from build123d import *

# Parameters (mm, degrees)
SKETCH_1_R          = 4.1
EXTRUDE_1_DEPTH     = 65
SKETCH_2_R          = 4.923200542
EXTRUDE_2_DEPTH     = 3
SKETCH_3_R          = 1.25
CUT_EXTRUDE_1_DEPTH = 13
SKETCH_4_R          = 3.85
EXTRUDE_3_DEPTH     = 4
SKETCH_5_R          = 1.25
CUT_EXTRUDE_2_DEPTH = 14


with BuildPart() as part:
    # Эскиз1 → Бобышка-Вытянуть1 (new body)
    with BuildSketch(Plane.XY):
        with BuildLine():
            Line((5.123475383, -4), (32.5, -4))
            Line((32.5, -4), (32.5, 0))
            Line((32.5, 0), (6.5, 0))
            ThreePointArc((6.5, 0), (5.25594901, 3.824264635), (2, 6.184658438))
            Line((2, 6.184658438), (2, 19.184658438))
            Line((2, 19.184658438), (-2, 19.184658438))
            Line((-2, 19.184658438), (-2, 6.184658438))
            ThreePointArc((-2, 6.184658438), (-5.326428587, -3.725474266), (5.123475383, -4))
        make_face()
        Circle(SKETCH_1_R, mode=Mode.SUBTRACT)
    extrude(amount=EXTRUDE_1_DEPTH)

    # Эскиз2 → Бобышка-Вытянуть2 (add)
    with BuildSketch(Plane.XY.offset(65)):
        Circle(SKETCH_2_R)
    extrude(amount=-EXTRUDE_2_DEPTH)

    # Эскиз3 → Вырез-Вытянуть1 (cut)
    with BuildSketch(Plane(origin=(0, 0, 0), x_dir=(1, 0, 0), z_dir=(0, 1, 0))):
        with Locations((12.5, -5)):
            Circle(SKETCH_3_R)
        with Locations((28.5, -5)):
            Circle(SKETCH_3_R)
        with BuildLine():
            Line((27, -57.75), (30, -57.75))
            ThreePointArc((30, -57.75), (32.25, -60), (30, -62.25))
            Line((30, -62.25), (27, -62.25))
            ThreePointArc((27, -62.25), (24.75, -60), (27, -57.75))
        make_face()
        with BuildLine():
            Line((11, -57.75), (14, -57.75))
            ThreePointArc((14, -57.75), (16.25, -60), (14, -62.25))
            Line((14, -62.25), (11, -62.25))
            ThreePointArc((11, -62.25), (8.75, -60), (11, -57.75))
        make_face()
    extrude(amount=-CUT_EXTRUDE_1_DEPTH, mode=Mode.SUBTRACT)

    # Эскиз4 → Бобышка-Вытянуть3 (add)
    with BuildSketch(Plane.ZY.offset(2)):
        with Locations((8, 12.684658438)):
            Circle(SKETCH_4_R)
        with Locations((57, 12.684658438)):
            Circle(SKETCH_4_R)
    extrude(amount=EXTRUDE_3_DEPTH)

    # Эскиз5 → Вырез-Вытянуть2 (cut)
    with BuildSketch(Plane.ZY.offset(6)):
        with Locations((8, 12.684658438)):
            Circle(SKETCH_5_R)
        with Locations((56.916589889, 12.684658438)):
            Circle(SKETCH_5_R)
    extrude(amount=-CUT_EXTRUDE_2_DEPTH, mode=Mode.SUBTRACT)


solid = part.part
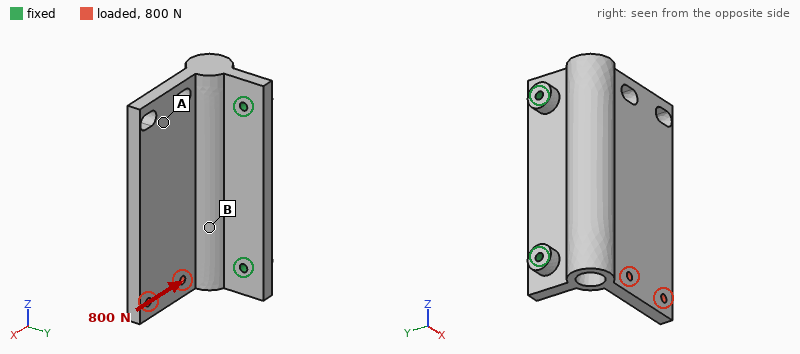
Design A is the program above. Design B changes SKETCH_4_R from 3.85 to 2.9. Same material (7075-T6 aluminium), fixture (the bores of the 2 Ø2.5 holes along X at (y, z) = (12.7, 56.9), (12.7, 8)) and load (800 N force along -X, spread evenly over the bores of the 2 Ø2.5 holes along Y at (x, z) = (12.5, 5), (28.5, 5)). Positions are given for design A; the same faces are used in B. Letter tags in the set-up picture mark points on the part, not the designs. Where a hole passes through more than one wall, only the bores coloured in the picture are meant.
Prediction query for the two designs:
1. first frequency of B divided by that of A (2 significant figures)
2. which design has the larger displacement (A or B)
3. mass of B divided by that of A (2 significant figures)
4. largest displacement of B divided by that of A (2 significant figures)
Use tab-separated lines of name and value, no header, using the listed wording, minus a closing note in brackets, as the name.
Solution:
first frequency of B divided by that of A	0.95
which design has the larger displacement	B
mass of B divided by that of A	0.99
largest displacement of B divided by that of A	1.1
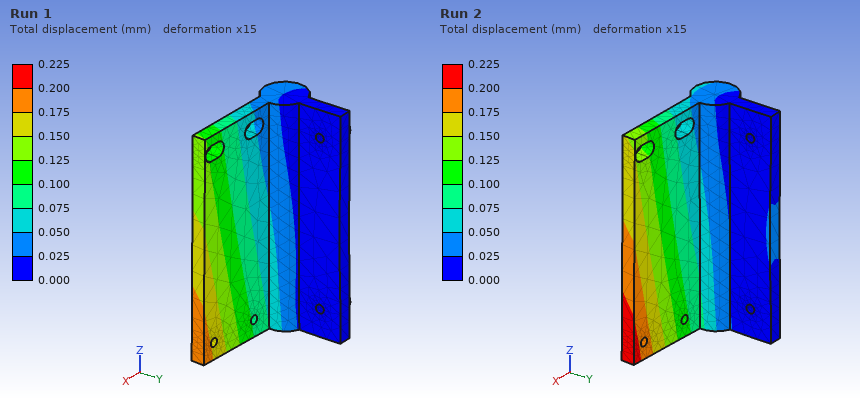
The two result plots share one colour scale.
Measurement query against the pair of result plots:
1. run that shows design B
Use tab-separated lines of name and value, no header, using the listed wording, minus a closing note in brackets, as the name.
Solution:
run that shows design B	Run 2
